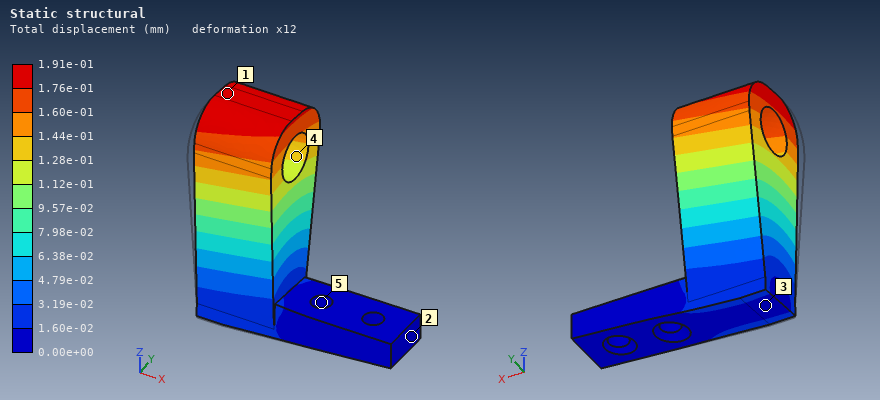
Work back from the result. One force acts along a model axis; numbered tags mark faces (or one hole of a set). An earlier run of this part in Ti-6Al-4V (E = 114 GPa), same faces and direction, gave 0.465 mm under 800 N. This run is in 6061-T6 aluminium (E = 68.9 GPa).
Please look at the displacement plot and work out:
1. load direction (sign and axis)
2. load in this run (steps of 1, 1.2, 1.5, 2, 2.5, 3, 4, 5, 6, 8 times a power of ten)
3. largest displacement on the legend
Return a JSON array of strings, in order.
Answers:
["+Y", "200 N", "1.91e-01 mm"]
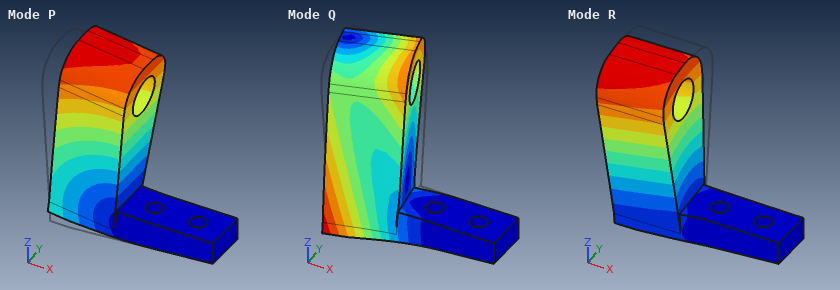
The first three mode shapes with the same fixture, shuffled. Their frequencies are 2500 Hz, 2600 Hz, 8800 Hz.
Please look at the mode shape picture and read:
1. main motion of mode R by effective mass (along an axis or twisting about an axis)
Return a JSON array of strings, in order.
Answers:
["along Y"]
